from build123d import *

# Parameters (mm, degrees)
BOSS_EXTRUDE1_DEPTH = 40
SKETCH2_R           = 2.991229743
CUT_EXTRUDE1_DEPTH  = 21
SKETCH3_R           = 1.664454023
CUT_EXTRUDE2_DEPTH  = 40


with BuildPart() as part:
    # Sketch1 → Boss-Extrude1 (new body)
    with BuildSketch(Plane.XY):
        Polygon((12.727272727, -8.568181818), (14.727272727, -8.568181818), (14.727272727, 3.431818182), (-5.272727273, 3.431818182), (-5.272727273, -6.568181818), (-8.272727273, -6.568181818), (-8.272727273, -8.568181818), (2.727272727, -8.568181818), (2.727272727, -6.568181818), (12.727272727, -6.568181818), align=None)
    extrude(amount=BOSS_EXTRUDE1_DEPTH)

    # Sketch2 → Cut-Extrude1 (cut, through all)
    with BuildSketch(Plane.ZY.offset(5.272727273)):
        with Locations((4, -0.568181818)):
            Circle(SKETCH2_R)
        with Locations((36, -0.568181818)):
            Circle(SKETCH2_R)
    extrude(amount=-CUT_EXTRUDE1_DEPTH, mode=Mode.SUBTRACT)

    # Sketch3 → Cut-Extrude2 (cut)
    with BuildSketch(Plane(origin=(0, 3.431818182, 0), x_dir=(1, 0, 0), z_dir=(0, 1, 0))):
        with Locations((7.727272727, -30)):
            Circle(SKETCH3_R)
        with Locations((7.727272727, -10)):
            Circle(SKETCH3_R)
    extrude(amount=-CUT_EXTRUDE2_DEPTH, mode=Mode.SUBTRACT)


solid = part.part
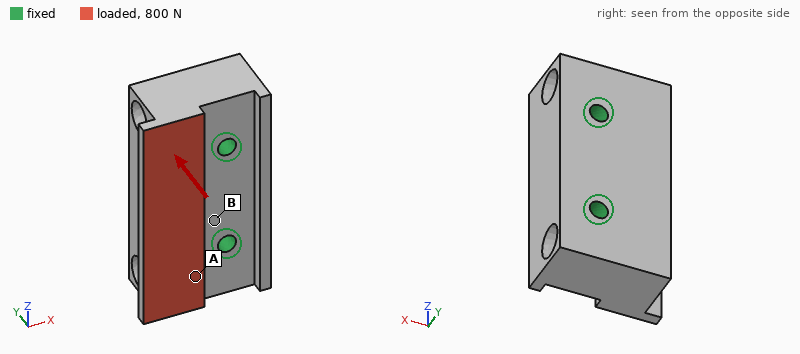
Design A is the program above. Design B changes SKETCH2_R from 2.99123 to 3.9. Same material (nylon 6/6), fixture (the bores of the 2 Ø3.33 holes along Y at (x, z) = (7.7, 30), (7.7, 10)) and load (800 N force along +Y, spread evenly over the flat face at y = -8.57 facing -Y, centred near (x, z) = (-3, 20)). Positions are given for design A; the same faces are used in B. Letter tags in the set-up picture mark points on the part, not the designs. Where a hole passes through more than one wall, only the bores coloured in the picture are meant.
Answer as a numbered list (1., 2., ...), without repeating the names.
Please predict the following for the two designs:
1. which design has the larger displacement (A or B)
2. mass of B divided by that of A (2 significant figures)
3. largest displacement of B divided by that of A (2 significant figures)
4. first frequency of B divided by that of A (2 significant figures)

1. B
2. 0.90
3. 1.3
4. 0.97
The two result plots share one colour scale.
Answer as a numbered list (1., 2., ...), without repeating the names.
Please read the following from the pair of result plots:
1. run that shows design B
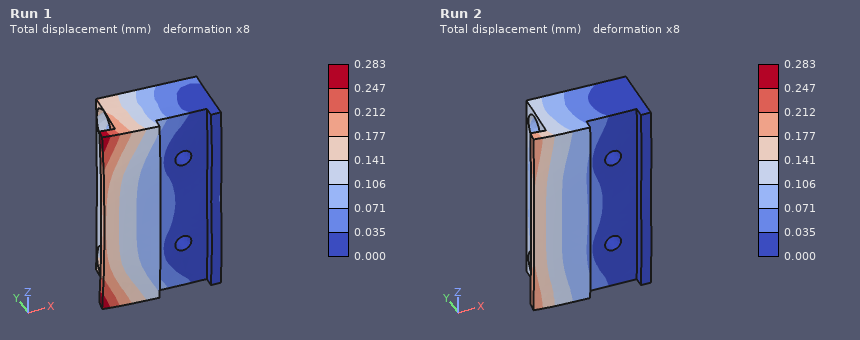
1. Run 1
